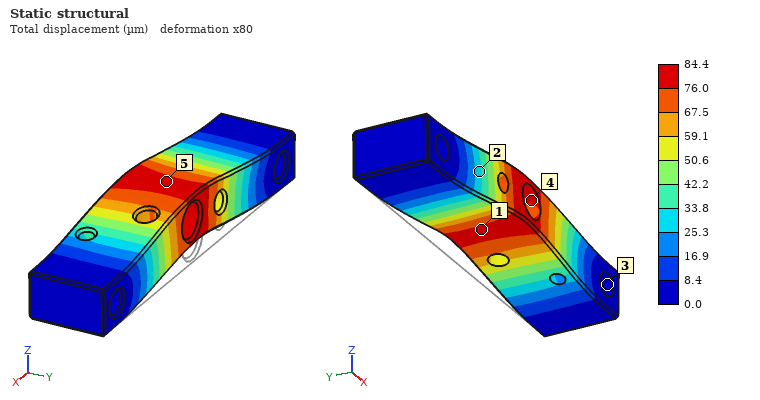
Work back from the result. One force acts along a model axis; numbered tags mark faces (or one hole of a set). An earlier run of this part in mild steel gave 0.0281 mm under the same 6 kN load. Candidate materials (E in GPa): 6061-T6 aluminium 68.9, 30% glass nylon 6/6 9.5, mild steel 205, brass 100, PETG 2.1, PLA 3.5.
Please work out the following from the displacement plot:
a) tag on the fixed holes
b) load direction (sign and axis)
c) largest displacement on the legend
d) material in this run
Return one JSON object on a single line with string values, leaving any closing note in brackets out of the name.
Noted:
{"tag on the fixed holes": "3", "load direction": "+Z", "largest displacement on the legend": "84.4 µm", "material in this run": "6061-T6 aluminium"}
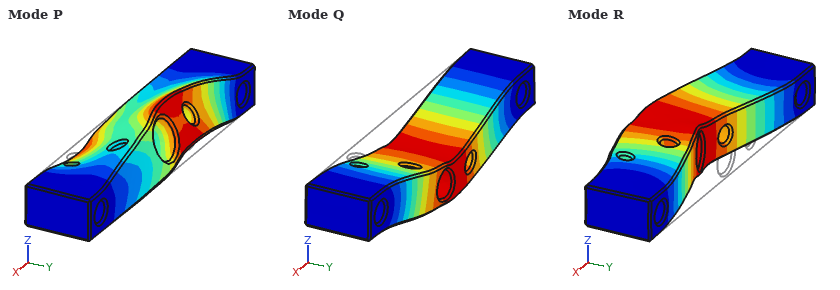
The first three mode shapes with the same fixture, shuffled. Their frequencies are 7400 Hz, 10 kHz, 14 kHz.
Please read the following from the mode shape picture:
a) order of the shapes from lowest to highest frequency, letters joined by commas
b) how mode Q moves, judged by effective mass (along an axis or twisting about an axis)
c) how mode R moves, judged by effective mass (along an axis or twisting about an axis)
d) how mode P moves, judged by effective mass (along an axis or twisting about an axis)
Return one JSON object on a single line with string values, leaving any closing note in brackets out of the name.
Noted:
{"order of the shapes from lowest to highest frequency, letters joined by commas": "Q, R, P", "how mode Q moves, judged by effective mass": "along Z", "how mode R moves, judged by effective mass": "along Y", "how mode P moves, judged by effective mass": "twisting about X"}
